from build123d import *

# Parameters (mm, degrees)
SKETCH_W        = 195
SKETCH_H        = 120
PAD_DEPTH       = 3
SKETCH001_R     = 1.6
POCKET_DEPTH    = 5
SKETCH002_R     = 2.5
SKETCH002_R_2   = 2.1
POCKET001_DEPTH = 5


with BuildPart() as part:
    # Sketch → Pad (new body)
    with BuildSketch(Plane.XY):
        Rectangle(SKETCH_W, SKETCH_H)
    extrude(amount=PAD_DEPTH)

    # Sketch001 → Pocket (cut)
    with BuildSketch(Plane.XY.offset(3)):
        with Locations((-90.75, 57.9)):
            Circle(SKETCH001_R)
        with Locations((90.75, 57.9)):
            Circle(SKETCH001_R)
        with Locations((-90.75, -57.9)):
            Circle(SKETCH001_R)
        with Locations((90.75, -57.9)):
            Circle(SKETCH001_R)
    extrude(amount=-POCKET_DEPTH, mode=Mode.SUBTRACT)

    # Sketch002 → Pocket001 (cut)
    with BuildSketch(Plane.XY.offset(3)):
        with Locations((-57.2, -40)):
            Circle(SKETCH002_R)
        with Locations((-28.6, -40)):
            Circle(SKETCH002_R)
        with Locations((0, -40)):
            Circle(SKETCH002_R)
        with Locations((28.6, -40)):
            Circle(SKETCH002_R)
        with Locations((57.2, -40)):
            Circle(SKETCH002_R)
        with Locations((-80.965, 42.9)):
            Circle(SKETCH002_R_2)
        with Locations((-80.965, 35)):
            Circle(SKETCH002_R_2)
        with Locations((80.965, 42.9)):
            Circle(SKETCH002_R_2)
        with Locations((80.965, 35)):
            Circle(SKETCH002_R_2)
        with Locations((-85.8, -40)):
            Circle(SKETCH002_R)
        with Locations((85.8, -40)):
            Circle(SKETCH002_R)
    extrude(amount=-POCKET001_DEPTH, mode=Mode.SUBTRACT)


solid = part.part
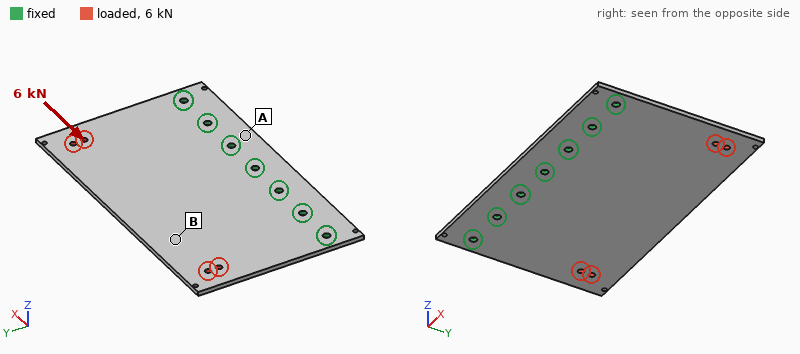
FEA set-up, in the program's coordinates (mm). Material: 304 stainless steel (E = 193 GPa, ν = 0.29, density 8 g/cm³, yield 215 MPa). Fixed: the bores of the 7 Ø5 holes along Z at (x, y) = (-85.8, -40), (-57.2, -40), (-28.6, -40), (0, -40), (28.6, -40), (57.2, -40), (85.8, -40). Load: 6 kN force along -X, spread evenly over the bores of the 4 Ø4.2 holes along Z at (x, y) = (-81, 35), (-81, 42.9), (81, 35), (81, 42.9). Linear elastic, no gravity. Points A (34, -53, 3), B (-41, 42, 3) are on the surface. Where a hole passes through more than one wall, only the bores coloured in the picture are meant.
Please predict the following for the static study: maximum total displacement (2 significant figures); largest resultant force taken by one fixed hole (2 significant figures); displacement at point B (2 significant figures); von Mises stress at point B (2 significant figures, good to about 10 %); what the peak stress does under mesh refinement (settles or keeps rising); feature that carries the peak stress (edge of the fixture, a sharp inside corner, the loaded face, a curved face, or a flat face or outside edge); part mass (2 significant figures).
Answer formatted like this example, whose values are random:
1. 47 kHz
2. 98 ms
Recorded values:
1. 22 µm
2. 2.3 kN
3. 15 µm
4. 16 MPa
5. keeps rising
6. edge of the fixture
7. 560 g
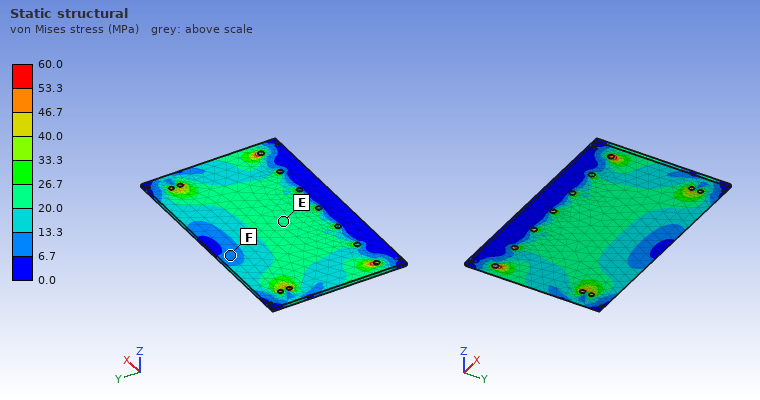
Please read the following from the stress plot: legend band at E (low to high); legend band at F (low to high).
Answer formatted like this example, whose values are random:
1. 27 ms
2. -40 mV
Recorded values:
1. 20.0 to 26.7 MPa
2. 6.7 to 13.3 MPa
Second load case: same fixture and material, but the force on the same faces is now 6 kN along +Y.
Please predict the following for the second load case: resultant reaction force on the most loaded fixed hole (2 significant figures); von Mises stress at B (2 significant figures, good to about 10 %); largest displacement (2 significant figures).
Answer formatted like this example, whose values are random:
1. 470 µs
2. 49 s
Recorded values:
1. 1.3 kN
2. 6.2 MPa
3. 11 µm
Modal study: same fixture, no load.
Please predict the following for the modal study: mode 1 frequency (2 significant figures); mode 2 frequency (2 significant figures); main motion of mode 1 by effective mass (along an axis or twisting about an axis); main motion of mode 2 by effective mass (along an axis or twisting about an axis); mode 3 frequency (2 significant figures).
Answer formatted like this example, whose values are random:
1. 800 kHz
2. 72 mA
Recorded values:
1. 250 Hz
2. 390 Hz
3. along Z
4. twisting about Y
5. 740 Hz
